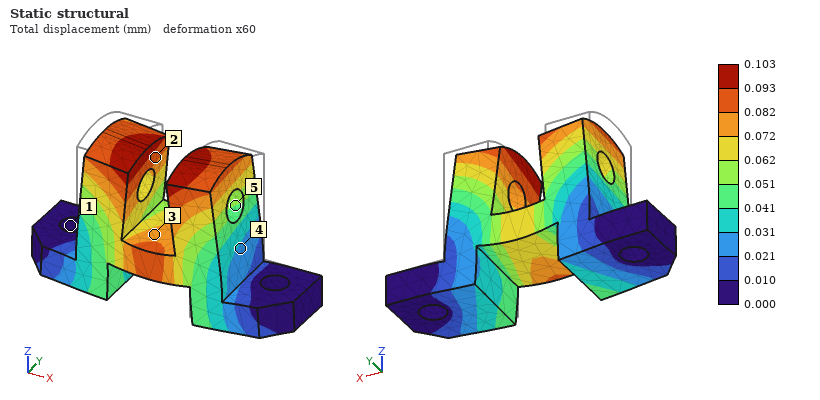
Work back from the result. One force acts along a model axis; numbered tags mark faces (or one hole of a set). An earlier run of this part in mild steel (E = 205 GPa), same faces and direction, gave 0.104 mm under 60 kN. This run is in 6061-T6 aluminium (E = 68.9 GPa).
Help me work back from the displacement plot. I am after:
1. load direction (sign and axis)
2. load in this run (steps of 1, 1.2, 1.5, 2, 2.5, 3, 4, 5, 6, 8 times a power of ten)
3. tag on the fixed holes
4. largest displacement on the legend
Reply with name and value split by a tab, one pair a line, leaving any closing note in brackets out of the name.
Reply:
load direction	-Z
load in this run	20 kN
tag on the fixed holes	1
largest displacement on the legend	0.103 mm
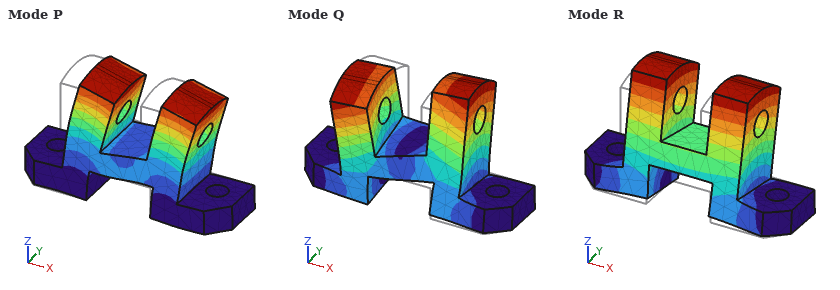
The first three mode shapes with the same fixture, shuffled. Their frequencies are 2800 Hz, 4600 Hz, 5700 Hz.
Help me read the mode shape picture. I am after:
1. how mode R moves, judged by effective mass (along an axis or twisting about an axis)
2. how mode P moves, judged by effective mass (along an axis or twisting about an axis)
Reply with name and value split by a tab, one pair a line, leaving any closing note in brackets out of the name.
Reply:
how mode R moves, judged by effective mass	along Y
how mode P moves, judged by effective mass	along X
